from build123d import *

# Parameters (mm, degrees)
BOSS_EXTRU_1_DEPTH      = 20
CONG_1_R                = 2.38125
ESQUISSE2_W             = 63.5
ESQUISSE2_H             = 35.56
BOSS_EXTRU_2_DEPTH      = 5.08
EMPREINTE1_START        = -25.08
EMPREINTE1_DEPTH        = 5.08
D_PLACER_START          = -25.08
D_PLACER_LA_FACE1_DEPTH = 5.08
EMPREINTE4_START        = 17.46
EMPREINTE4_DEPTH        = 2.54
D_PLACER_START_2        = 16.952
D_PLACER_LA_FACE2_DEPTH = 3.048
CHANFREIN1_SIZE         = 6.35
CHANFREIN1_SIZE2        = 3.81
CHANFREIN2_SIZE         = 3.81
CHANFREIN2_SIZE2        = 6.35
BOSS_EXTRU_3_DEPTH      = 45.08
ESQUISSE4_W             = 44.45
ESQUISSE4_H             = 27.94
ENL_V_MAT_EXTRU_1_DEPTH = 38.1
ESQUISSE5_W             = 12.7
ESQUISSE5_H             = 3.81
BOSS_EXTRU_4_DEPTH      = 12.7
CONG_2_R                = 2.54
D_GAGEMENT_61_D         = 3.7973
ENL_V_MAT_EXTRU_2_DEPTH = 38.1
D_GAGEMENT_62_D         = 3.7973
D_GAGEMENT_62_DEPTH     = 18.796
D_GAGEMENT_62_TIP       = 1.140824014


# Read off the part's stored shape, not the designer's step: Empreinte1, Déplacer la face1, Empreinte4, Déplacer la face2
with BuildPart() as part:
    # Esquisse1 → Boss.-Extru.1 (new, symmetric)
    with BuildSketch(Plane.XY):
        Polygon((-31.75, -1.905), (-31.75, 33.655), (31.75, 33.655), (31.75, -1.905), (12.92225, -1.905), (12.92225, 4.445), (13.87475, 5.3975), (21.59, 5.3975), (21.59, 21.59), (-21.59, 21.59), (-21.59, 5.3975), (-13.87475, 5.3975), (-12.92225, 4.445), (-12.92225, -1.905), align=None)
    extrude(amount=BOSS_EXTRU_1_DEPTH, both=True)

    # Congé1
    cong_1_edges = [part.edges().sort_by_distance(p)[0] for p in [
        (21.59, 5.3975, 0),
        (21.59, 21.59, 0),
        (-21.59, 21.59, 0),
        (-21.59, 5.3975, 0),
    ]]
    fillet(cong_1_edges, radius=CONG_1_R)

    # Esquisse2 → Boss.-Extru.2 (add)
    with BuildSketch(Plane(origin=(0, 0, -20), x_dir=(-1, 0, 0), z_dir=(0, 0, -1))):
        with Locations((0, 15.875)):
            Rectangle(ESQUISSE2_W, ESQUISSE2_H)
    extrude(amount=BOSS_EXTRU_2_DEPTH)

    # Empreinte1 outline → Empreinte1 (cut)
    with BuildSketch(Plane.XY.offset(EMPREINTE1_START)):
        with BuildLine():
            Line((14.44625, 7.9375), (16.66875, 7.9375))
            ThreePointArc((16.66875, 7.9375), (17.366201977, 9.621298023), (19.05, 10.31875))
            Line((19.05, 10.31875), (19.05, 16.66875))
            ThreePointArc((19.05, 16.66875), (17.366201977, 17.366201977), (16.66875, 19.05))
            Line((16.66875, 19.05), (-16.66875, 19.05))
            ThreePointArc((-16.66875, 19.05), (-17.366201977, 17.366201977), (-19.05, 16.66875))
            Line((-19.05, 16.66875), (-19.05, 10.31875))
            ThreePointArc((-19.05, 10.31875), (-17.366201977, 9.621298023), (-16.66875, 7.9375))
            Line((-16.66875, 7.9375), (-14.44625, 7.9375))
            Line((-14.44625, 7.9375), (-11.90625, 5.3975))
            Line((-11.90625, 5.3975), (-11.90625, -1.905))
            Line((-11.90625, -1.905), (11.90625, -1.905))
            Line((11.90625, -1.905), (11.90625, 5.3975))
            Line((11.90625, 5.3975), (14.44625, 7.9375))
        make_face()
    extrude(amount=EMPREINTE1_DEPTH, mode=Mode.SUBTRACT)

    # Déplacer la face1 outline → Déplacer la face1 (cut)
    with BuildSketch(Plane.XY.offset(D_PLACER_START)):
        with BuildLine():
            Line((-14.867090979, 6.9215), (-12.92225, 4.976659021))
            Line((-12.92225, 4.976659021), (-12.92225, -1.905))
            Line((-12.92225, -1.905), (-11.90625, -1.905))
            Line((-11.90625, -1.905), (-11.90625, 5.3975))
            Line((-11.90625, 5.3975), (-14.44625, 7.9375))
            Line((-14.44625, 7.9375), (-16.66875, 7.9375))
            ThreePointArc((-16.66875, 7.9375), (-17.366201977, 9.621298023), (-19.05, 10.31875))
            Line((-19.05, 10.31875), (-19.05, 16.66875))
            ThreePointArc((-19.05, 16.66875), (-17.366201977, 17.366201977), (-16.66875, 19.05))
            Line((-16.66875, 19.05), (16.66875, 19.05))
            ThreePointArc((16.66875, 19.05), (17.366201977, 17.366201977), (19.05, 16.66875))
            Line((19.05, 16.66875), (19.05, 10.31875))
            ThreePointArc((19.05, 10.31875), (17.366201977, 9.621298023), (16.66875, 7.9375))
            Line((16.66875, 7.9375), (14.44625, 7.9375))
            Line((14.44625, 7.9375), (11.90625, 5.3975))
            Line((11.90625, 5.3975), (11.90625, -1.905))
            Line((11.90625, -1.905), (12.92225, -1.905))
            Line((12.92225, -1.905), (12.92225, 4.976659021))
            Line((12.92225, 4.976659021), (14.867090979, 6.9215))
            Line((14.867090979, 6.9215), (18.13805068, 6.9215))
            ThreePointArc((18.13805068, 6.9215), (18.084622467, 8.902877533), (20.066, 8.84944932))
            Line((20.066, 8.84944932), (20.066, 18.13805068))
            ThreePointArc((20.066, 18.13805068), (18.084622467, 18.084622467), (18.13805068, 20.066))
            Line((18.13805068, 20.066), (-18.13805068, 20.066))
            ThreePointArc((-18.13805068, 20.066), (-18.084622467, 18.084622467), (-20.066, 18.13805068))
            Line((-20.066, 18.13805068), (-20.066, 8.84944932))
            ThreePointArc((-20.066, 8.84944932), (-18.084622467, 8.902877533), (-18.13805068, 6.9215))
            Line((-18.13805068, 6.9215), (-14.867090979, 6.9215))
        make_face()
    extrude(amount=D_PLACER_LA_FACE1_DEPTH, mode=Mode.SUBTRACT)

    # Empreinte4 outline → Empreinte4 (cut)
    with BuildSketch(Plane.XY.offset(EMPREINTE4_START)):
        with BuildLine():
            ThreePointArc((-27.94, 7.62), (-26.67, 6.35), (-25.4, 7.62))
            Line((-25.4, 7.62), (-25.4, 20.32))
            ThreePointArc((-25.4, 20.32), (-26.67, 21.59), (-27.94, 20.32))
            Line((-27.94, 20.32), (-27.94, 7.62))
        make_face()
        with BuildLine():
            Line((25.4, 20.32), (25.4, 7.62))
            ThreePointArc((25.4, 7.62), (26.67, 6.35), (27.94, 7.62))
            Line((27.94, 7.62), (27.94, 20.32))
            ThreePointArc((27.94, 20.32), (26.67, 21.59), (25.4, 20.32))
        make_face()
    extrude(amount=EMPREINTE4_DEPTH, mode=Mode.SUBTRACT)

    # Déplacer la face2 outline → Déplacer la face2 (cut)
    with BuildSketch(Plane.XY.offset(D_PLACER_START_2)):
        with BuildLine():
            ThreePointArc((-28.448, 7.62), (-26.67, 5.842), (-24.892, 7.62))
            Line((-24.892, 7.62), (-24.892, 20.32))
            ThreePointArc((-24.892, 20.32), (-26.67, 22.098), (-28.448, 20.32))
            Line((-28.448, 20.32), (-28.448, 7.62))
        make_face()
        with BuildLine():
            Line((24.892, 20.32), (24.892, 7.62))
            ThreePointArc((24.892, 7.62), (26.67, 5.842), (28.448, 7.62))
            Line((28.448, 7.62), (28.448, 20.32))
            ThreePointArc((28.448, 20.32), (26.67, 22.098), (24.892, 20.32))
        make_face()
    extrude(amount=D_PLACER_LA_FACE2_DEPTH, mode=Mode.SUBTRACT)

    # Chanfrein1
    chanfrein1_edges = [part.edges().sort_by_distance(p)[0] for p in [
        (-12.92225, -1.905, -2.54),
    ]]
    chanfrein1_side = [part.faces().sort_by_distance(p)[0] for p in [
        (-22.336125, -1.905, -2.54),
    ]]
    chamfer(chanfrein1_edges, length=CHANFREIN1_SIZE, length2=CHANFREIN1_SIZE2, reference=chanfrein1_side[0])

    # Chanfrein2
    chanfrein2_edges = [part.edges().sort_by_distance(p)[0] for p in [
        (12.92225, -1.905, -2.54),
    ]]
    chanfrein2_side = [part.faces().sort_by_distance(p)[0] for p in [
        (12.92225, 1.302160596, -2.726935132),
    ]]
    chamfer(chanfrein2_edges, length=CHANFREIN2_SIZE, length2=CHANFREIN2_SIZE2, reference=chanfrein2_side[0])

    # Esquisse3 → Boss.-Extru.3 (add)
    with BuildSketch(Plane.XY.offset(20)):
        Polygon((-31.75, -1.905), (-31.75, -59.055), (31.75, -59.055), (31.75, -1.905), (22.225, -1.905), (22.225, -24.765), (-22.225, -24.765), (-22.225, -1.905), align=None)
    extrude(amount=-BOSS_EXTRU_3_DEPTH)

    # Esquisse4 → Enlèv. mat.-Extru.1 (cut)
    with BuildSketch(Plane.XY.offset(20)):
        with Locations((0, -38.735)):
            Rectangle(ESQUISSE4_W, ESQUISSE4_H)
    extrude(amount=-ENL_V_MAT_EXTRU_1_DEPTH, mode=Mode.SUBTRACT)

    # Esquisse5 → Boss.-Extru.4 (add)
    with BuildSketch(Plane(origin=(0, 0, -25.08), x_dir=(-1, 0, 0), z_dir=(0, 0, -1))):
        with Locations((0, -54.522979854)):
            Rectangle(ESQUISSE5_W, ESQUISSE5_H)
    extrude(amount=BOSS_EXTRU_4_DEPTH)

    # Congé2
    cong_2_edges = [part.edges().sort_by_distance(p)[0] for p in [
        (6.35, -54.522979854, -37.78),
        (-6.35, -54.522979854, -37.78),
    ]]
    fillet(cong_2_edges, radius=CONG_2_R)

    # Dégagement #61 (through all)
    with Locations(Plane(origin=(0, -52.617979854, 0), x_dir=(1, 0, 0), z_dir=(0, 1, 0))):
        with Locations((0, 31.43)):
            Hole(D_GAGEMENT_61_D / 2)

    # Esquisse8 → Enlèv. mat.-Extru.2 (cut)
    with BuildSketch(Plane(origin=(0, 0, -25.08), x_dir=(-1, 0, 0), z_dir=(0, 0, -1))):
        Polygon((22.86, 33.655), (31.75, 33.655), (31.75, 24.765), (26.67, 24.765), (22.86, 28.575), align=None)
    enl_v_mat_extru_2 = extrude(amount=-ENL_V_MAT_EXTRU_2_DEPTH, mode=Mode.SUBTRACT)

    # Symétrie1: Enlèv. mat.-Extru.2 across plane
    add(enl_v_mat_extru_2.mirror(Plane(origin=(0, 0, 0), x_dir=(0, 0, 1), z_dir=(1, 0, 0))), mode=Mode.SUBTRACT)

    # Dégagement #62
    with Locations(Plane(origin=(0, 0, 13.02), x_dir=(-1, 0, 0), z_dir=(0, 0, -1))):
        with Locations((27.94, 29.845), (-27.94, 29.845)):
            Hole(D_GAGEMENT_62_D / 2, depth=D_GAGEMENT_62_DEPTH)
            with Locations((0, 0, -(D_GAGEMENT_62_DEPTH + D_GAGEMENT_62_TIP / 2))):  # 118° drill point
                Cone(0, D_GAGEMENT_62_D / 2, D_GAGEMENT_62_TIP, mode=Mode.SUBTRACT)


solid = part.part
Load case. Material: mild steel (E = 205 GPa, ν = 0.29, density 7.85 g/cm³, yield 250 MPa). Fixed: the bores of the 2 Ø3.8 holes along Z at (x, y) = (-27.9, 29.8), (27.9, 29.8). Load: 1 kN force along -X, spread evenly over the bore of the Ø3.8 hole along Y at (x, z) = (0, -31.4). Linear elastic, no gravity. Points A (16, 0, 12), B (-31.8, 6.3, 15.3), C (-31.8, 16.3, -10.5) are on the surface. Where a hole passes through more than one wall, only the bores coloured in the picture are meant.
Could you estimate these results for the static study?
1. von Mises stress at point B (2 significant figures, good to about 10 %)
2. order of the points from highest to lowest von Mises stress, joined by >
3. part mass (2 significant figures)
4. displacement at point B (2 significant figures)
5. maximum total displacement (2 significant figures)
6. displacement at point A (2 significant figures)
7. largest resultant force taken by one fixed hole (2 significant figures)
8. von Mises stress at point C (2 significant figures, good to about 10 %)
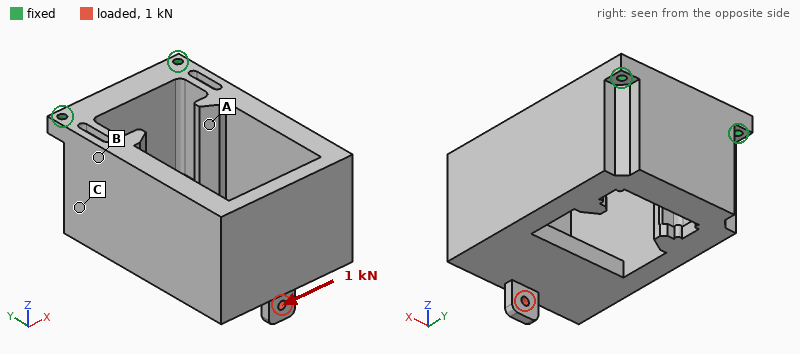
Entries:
16 MPa
B > C > A
990 g
8.2 µm
39 µm
12 µm
1.8 kN
9.9 MPa
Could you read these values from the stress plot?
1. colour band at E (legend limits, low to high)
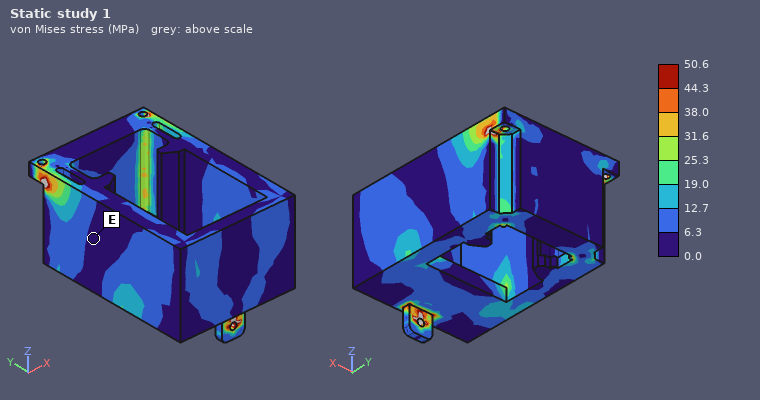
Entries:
0.0 to 6.3 MPa
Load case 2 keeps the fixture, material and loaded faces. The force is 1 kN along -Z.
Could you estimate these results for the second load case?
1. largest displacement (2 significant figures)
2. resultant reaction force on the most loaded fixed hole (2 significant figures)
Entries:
0.32 mm
710 N
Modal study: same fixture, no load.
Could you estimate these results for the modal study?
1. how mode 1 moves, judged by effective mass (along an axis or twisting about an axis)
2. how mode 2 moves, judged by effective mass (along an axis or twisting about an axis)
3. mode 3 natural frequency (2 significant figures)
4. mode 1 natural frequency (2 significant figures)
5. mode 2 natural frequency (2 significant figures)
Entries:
along Z
along X
2700 Hz
460 Hz
1100 Hz
